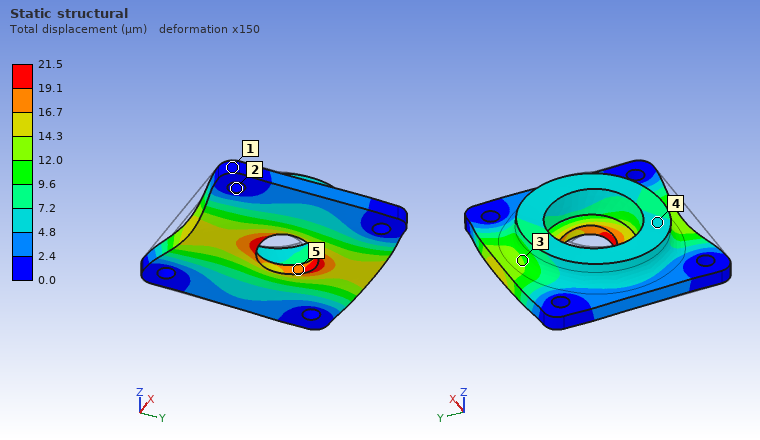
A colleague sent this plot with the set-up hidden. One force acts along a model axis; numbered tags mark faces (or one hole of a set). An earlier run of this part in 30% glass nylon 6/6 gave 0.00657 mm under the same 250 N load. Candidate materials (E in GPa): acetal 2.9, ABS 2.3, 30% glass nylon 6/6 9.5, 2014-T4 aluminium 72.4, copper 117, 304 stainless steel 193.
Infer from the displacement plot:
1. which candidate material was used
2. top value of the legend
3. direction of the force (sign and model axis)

acetal
21.5 µm
+Y
